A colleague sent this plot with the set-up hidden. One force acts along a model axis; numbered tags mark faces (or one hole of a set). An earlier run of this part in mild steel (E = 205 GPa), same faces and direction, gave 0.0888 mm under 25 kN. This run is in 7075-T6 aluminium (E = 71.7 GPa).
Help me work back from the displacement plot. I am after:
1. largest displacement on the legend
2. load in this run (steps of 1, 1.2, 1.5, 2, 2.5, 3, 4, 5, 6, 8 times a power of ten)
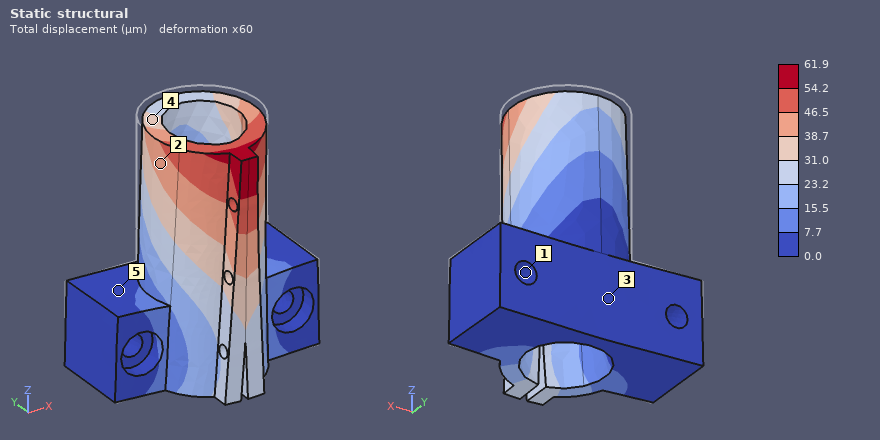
61.9 µm
6 kN
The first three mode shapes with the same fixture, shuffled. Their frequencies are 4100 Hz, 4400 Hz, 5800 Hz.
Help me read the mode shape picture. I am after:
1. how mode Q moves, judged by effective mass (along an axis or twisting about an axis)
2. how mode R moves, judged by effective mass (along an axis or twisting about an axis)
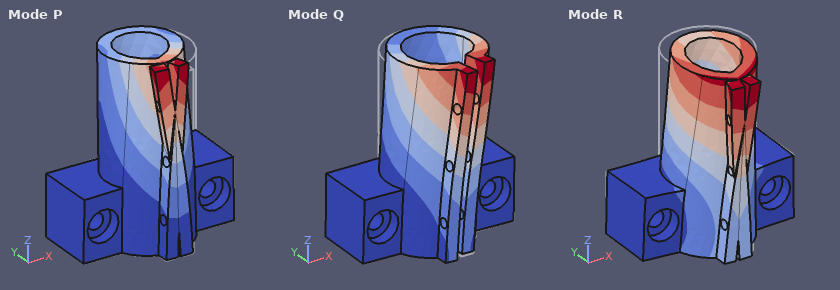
along X
along Y
